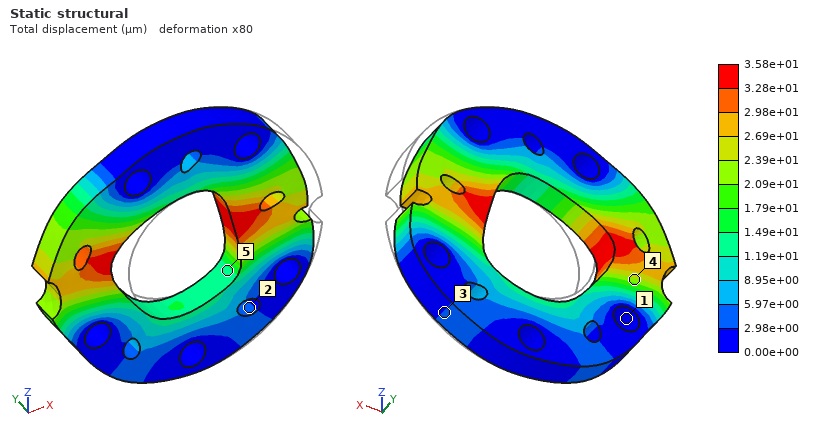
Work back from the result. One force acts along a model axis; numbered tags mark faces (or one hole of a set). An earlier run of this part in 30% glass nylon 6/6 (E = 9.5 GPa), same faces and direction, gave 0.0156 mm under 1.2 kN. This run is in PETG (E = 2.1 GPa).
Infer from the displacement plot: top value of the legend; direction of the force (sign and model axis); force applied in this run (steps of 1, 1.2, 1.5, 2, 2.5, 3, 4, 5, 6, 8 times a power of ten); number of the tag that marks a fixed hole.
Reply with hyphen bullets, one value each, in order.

- 3.58e+01 µm
- -X
- 600 N
- 1
